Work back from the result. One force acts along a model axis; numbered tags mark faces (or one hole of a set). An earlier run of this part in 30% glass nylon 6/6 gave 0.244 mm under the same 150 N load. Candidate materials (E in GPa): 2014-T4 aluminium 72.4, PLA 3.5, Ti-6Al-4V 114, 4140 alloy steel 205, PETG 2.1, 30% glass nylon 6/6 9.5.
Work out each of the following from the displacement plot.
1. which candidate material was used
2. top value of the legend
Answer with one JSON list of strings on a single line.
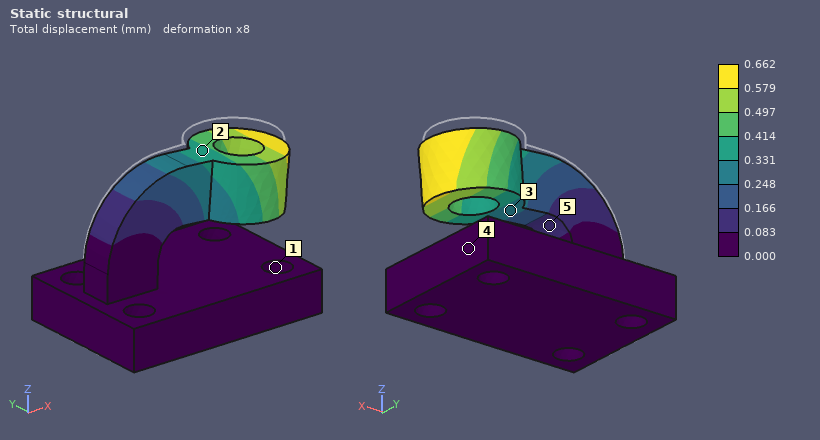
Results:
["PLA", "0.662 mm"]
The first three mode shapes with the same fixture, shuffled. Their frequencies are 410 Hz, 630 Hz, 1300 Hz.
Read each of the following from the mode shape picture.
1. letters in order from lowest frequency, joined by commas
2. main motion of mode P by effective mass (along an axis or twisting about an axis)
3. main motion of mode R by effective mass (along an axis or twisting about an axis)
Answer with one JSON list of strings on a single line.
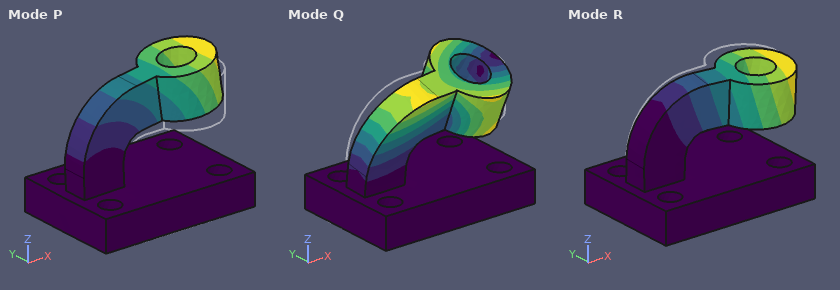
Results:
["R, P, Q", "along Z", "along Y"]
